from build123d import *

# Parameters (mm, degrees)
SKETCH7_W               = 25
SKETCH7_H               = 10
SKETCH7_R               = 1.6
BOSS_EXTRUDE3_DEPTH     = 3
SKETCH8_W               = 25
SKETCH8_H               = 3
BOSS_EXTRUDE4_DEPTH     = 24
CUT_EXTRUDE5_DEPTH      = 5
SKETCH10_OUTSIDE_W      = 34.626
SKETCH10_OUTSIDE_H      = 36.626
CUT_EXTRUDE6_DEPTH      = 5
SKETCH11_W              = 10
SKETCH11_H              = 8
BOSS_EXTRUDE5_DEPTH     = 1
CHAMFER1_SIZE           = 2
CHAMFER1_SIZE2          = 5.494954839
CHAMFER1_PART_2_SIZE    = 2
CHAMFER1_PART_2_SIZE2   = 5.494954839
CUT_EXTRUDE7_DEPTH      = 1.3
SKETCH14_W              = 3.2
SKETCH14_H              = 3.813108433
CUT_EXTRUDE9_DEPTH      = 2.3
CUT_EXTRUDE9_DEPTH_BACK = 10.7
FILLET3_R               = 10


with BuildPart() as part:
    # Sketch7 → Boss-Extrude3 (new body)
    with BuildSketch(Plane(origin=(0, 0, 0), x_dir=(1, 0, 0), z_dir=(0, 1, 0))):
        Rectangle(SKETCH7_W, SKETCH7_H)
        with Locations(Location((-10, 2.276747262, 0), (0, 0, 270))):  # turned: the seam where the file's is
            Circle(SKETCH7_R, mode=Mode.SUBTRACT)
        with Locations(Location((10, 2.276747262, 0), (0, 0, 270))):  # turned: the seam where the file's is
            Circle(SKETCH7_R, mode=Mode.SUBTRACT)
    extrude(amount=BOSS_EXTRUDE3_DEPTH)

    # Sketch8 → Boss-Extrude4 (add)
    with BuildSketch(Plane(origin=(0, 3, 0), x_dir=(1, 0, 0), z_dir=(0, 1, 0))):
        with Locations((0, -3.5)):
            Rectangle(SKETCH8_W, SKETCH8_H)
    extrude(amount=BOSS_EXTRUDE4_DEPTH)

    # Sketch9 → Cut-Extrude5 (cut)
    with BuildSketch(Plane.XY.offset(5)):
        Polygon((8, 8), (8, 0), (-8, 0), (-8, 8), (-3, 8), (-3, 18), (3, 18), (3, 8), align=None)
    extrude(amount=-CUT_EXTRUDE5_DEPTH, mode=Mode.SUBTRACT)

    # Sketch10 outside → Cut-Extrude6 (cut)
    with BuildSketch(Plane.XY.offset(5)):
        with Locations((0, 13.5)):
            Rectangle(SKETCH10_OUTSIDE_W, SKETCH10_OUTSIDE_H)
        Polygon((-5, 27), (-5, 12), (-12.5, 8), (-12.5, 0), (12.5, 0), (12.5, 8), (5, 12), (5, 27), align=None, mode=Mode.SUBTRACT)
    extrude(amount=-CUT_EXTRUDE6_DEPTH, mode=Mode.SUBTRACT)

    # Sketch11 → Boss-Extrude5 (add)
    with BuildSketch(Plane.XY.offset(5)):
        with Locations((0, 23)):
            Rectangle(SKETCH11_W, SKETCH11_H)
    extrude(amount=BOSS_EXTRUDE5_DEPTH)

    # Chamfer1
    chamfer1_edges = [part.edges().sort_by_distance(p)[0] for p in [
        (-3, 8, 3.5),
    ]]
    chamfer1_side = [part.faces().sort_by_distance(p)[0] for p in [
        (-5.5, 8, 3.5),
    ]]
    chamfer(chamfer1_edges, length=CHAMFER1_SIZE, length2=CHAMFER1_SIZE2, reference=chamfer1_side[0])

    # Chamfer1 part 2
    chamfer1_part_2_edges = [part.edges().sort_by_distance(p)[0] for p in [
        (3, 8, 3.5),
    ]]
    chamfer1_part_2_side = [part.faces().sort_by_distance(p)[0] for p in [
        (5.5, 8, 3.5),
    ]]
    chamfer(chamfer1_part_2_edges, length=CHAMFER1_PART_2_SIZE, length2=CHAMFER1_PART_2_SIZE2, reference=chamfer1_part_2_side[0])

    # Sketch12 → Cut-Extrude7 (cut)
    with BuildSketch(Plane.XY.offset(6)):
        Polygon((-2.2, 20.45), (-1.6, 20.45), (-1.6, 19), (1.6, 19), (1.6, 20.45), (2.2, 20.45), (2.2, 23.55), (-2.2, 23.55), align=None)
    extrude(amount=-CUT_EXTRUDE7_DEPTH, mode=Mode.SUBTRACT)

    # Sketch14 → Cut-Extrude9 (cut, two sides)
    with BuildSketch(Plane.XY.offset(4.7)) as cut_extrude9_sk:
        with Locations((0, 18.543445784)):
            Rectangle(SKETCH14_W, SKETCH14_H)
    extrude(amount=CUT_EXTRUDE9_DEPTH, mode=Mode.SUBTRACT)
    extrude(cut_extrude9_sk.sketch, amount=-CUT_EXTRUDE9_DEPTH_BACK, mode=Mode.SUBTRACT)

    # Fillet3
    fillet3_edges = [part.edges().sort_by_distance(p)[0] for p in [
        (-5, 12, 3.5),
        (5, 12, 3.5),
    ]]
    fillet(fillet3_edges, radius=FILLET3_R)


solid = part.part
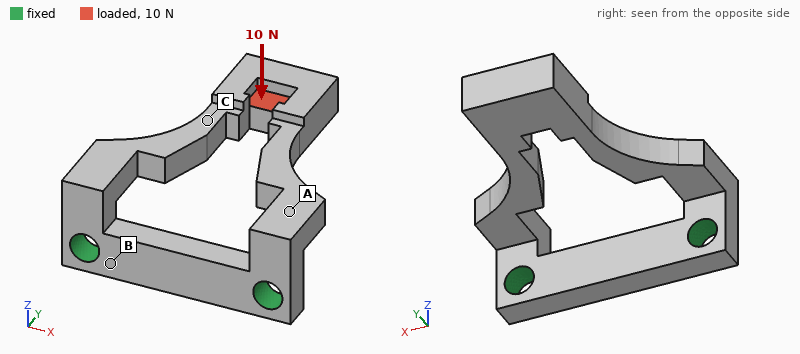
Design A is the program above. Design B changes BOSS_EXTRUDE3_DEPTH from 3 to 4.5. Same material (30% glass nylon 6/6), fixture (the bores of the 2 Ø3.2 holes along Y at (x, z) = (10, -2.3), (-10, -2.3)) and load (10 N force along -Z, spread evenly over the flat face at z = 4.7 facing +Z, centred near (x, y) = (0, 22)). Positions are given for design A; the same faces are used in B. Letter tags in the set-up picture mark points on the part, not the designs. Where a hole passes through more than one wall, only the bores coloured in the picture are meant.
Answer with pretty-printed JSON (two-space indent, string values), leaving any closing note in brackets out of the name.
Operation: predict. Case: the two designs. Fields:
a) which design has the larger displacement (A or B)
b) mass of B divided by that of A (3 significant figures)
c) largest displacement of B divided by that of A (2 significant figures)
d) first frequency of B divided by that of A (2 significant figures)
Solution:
{
  "which design has the larger displacement": "A",
  "mass of B divided by that of A": "1.17",
  "largest displacement of B divided by that of A": "0.75",
  "first frequency of B divided by that of A": "1.2"
}
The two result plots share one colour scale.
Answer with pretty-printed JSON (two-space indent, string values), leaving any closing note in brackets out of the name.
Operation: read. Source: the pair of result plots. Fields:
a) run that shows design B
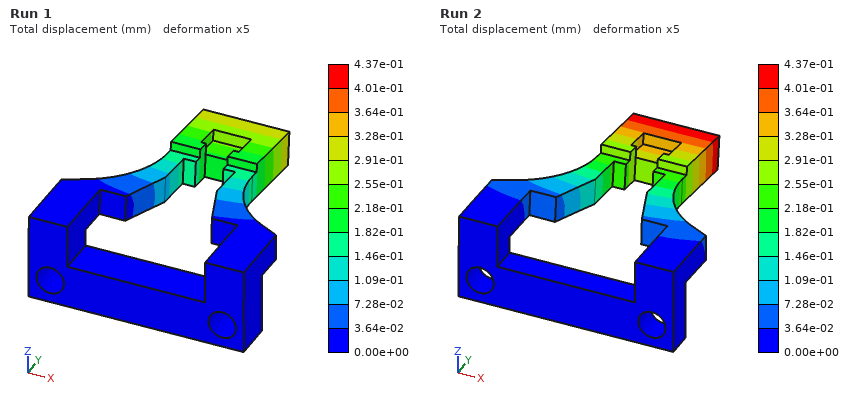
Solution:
{
  "run that shows design B": "Run 1"
}
